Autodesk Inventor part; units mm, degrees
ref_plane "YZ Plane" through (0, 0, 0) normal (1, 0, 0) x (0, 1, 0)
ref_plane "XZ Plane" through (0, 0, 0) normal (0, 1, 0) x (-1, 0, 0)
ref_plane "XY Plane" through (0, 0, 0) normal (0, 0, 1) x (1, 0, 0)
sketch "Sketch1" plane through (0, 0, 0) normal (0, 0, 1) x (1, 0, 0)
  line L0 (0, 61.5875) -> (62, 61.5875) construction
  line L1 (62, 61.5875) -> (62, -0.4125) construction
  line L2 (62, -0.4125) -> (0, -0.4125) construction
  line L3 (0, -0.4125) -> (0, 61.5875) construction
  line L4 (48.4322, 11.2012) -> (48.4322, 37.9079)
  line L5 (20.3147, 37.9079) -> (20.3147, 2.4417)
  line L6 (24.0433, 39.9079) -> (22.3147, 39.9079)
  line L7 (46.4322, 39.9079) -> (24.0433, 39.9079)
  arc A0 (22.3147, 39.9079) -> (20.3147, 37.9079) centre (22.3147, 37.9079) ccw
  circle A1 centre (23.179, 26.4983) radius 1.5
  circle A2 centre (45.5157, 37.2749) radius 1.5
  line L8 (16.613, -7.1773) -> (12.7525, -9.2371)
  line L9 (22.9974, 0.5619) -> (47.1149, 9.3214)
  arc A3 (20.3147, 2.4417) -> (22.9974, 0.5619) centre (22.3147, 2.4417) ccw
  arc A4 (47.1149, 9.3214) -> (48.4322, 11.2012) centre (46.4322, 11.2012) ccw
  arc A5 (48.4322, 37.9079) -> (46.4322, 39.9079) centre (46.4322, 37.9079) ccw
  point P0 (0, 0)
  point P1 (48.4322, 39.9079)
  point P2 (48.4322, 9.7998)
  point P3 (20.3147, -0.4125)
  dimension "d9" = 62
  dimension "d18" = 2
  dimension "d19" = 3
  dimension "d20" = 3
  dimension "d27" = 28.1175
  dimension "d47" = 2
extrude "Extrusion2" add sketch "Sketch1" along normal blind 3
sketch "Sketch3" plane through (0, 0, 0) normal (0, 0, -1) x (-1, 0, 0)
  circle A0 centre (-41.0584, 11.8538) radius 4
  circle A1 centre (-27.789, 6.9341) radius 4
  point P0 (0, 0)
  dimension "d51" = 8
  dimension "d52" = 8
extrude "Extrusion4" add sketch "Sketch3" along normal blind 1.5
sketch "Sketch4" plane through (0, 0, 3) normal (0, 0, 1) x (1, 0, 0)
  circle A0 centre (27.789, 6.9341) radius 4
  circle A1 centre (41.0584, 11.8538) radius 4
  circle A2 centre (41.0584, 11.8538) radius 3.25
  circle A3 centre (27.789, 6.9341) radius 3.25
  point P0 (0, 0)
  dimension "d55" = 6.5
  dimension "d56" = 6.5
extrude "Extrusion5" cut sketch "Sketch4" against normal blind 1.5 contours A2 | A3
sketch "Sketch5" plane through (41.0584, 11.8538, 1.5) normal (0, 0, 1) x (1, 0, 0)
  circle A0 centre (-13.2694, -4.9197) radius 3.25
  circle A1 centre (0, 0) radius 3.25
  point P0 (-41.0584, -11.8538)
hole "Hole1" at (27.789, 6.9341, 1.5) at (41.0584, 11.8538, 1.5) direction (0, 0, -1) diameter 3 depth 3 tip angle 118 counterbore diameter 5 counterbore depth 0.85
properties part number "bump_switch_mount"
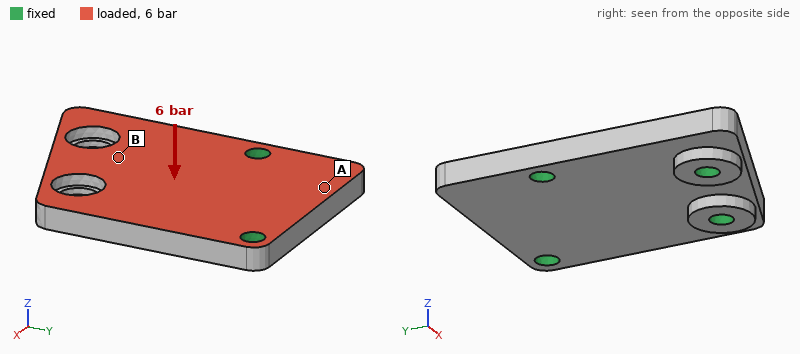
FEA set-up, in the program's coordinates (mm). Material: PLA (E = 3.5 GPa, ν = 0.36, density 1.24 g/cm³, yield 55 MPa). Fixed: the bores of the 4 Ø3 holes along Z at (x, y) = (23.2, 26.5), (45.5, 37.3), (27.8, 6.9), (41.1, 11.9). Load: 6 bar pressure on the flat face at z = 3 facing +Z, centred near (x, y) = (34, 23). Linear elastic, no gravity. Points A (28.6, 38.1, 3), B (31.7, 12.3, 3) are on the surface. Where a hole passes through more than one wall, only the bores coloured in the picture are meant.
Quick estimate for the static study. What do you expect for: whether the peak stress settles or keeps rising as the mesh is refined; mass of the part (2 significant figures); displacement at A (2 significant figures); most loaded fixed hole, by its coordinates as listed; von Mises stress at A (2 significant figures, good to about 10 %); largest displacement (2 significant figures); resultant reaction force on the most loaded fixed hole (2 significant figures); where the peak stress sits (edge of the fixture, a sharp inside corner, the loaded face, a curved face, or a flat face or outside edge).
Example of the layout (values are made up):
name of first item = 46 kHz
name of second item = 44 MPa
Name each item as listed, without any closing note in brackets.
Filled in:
whether the peak stress settles or keeps rising as the mesh is refined = keeps rising
mass of the part = 3.6 g
displacement at A = 0.17 mm
most loaded fixed hole, by its coordinates as listed = (23.2, 26.5)
von Mises stress at A = 8.5 MPa
largest displacement = 0.21 mm
resultant reaction force on the most loaded fixed hole = 190 N
where the peak stress sits = edge of the fixture
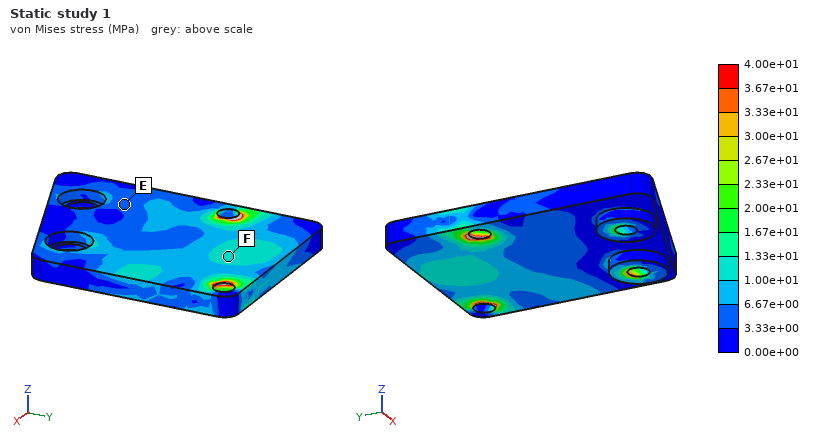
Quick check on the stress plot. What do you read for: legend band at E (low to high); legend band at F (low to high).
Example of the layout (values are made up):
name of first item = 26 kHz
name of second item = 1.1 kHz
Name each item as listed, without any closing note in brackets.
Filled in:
legend band at E = 3.33e+00 to 6.67e+00 MPa
legend band at F = 1.00e+01 to 1.33e+01 MPa
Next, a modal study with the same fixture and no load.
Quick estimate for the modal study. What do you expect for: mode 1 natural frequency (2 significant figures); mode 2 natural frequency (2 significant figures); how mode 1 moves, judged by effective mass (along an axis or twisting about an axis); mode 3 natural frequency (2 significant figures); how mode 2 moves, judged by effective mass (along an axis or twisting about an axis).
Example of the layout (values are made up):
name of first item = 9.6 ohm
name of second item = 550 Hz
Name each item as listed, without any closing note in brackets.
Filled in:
mode 1 natural frequency = 5600 Hz
mode 2 natural frequency = 7400 Hz
how mode 1 moves, judged by effective mass = along Z
mode 3 natural frequency = 9800 Hz
how mode 2 moves, judged by effective mass = along Z
